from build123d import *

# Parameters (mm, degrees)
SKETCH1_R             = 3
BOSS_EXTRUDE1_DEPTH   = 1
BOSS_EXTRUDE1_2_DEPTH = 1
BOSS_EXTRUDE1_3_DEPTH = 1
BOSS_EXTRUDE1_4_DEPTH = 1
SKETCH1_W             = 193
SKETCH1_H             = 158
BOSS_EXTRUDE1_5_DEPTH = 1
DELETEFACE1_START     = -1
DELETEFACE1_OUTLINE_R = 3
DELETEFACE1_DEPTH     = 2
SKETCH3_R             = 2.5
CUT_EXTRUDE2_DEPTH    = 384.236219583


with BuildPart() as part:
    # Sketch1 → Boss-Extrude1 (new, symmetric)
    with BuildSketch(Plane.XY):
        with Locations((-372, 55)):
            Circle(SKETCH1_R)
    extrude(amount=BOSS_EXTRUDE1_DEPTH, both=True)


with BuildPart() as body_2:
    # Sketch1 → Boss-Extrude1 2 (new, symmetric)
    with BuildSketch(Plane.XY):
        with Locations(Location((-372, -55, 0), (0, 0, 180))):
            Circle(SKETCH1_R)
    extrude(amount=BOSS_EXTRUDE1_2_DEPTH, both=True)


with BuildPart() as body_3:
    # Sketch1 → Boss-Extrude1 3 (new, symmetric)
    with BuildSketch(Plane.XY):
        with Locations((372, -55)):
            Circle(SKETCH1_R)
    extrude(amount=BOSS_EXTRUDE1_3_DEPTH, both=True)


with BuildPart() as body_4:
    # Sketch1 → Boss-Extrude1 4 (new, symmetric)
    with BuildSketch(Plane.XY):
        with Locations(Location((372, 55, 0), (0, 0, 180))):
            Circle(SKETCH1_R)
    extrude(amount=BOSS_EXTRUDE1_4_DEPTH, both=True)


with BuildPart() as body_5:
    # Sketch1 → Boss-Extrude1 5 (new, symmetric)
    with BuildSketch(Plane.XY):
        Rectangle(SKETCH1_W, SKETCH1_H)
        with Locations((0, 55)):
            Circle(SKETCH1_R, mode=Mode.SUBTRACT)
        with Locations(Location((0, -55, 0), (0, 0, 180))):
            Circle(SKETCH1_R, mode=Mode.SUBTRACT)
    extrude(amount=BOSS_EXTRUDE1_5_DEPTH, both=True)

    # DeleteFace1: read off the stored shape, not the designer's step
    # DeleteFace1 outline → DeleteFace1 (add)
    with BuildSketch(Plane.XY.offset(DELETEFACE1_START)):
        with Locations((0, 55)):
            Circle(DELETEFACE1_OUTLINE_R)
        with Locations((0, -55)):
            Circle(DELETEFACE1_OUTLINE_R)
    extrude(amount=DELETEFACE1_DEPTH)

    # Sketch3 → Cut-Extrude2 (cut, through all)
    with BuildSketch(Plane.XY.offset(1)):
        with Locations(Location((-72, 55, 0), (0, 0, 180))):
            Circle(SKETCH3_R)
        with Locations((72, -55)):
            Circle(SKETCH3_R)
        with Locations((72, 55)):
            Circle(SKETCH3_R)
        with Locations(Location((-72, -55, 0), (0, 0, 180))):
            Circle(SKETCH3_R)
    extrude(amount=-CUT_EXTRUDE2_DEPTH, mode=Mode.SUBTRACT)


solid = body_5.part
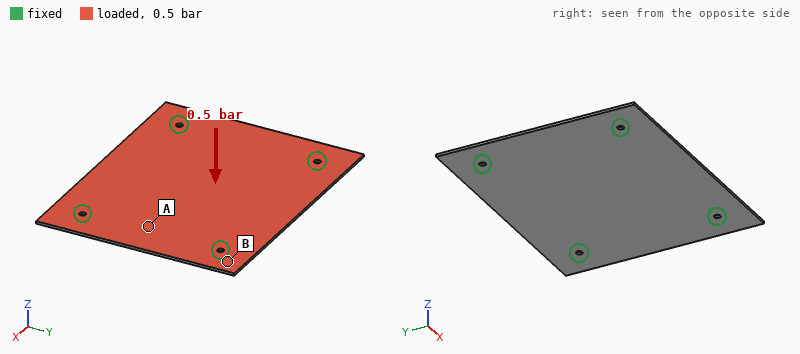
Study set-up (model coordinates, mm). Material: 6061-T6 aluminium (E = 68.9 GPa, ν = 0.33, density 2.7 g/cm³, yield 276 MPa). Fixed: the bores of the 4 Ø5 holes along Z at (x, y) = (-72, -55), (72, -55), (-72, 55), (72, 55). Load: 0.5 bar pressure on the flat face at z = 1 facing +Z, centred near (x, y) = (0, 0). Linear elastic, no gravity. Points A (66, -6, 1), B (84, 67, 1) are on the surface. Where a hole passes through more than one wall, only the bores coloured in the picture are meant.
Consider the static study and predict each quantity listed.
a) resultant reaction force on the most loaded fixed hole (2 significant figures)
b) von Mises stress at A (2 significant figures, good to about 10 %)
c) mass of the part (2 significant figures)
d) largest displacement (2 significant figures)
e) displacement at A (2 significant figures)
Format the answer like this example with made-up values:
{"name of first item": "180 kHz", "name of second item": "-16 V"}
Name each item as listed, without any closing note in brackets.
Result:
{"resultant reaction force on the most loaded fixed hole": "380 N", "von Mises stress at A": "52 MPa", "mass of the part": "160 g", "largest displacement": "1.9 mm", "displacement at A": "0.75 mm"}
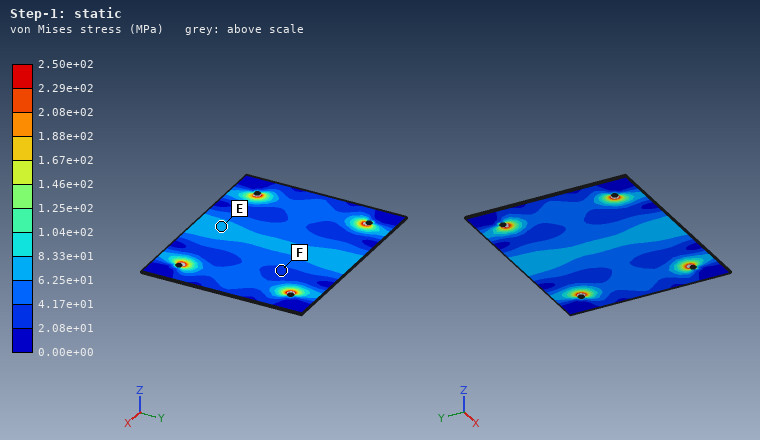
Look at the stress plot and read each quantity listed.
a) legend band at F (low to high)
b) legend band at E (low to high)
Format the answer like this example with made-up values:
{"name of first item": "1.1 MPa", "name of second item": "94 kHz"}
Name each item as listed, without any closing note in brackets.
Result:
{"legend band at F": "2.08e+01 to 4.17e+01 MPa", "legend band at E": "6.25e+01 to 8.33e+01 MPa"}
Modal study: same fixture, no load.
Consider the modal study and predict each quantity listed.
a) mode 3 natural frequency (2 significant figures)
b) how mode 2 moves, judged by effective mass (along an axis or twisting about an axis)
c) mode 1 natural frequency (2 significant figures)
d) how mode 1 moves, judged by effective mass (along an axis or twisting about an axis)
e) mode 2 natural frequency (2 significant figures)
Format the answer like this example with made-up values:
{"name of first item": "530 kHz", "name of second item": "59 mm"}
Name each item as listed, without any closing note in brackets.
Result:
{"mode 3 natural frequency": "710 Hz", "how mode 2 moves, judged by effective mass": "twisting about X", "mode 1 natural frequency": "410 Hz", "how mode 1 moves, judged by effective mass": "along Z", "mode 2 natural frequency": "560 Hz"}
